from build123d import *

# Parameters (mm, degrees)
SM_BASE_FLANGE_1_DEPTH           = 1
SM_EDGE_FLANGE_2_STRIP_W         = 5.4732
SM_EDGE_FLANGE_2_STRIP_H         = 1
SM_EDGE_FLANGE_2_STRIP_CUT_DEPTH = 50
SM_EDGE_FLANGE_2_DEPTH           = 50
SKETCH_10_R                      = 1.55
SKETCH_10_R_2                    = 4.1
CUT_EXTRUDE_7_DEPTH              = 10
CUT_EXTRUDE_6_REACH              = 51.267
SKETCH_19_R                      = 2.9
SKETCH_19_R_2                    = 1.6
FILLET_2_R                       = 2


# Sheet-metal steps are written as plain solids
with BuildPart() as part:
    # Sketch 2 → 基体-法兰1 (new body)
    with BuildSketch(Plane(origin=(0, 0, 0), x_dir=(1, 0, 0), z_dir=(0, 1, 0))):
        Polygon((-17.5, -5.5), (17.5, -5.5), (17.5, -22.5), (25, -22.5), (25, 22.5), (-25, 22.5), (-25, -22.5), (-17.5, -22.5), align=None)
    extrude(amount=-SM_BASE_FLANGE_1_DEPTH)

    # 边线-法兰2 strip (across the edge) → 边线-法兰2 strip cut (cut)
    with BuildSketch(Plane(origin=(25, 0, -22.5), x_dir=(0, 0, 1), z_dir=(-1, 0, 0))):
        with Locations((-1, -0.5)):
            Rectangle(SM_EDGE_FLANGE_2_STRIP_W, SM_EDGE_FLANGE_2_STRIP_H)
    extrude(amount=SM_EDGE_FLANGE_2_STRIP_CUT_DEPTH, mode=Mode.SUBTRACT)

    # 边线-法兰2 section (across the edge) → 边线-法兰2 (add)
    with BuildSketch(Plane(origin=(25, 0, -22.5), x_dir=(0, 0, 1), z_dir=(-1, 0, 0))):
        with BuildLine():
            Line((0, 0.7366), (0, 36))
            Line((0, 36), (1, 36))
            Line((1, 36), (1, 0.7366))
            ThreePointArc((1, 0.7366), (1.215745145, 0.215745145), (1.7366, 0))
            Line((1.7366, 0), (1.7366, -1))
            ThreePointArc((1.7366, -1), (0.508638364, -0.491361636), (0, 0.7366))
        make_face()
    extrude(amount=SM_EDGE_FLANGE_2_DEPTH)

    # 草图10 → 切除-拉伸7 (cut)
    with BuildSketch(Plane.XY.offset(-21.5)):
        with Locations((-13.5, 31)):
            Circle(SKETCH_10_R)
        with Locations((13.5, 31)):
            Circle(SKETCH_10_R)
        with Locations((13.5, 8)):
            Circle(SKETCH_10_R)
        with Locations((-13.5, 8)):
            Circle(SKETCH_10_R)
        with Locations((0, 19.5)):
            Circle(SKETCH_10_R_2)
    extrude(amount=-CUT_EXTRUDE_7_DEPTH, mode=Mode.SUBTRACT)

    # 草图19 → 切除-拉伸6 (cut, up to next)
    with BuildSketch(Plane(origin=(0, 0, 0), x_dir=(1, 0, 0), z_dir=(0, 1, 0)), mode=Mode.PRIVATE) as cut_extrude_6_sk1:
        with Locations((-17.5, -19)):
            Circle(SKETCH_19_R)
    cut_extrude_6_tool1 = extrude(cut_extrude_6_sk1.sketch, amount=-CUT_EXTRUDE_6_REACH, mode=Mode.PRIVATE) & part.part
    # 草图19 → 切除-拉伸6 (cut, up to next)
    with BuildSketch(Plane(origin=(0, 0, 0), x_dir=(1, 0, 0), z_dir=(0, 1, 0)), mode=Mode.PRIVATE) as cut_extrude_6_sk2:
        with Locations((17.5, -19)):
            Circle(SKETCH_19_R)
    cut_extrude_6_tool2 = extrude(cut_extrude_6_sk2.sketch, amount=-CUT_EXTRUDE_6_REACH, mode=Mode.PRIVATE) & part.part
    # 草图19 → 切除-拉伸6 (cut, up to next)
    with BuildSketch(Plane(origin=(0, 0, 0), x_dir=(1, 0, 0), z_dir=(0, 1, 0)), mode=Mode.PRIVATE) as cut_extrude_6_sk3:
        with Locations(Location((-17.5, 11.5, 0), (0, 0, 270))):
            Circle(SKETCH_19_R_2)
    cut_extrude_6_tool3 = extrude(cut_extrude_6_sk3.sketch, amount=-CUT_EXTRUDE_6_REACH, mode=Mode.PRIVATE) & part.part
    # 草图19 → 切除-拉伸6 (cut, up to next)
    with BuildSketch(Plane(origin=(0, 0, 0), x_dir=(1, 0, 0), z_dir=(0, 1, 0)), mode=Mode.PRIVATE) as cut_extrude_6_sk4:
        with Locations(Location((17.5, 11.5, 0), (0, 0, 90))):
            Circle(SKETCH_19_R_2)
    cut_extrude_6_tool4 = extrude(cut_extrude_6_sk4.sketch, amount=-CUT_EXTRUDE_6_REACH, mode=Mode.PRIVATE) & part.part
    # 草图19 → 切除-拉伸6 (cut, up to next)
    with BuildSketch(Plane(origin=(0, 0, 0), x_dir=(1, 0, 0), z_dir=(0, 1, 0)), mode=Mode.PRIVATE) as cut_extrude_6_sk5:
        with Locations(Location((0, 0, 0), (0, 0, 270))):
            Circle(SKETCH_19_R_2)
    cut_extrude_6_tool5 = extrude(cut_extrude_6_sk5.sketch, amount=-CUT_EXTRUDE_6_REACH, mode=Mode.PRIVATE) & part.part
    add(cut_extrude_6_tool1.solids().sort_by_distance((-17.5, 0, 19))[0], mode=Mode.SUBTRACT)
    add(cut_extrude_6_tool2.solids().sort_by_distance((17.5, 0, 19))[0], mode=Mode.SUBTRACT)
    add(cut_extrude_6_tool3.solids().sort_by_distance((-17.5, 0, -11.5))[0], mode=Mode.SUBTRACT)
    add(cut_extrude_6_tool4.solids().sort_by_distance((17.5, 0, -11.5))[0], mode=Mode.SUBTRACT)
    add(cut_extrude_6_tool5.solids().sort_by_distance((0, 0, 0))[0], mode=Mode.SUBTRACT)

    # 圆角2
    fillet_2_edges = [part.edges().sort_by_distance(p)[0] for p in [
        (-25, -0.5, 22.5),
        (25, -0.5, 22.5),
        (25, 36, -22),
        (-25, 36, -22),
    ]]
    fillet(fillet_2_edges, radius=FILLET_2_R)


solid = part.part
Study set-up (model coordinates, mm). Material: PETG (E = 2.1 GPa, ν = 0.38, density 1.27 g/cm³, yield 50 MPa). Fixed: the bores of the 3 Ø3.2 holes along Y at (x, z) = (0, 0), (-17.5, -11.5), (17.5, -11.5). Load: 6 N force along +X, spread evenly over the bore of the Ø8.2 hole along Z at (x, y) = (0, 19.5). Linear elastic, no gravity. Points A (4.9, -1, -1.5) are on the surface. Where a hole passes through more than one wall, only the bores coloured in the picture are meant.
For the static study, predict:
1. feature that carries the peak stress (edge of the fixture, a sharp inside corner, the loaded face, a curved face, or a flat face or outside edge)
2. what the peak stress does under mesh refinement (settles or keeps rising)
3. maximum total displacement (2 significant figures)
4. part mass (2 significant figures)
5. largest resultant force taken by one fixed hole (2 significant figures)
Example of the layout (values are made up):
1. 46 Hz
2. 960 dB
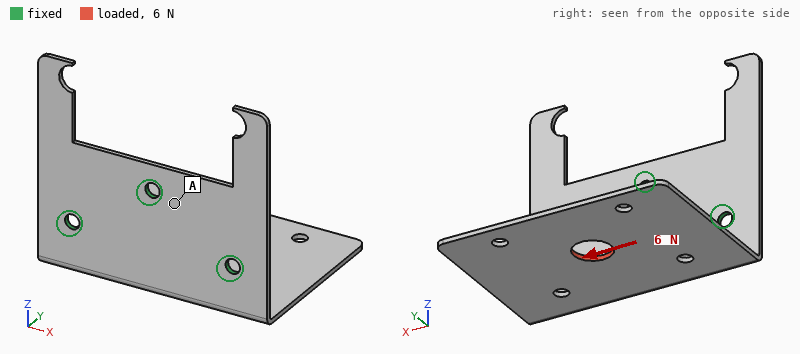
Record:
1. edge of the fixture
2. keeps rising
3. 0.73 mm
4. 4.2 g
5. 4.7 N
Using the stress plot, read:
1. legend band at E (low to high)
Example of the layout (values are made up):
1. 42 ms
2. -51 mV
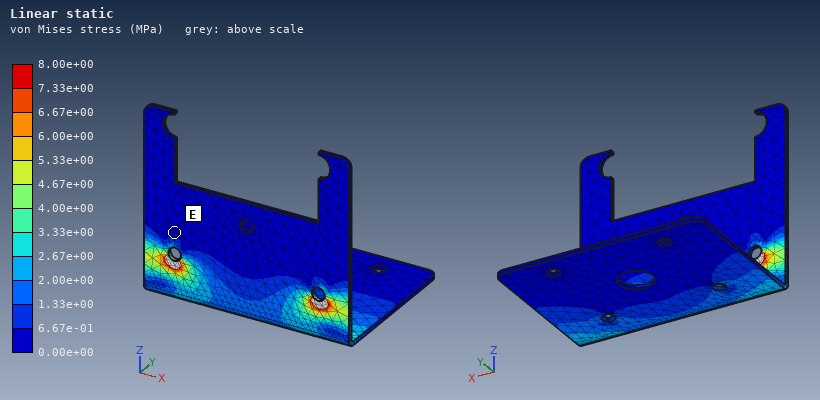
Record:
1. 0.00e+00 to 6.67e-01 MPa
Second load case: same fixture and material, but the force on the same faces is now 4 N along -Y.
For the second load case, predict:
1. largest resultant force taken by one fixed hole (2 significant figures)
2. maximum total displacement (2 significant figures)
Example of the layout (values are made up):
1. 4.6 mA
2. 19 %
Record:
1. 2.2 N
2. 0.89 mm
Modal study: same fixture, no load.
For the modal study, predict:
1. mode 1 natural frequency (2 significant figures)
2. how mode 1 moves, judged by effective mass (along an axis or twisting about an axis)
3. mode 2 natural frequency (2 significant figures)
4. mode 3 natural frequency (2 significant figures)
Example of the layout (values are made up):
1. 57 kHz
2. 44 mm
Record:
1. 110 Hz
2. along Z
3. 250 Hz
4. 330 Hz
